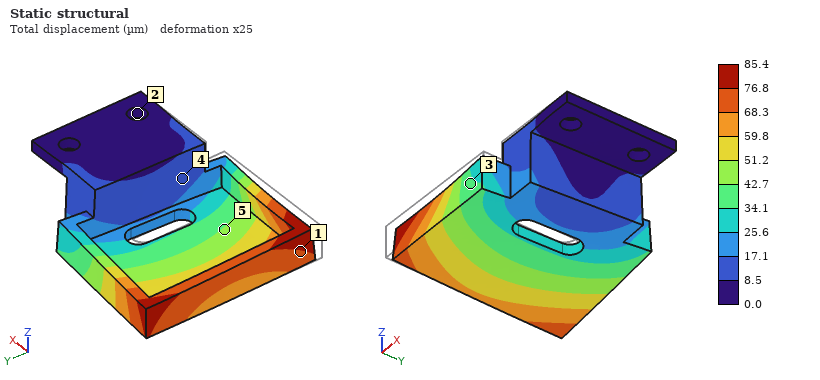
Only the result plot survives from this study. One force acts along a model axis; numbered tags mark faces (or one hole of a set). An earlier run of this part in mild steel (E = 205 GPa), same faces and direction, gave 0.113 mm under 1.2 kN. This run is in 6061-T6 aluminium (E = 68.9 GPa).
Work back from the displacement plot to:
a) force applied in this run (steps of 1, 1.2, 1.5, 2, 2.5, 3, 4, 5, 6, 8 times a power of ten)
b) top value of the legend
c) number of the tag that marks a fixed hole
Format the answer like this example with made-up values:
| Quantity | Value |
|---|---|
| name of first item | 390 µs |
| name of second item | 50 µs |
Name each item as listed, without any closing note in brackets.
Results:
| Quantity | Value |
|---|---|
| force applied in this run | 300 N |
| top value of the legend | 85.4 µm |
| number of the tag that marks a fixed hole | 2 |
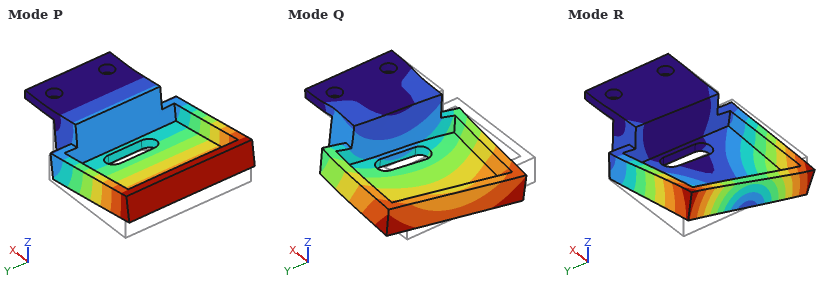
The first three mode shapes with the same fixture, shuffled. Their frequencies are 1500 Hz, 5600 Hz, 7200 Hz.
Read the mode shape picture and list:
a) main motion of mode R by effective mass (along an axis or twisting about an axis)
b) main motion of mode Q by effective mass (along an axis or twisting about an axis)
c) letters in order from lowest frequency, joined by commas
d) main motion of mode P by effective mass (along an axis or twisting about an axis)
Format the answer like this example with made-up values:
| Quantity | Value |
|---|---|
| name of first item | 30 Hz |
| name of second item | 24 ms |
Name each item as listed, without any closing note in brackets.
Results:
| Quantity | Value |
|---|---|
| main motion of mode R by effective mass | twisting about X |
| main motion of mode Q by effective mass | along Y |
| letters in order from lowest frequency, joined by commas | P, R, Q |
| main motion of mode P by effective mass | along Z |
